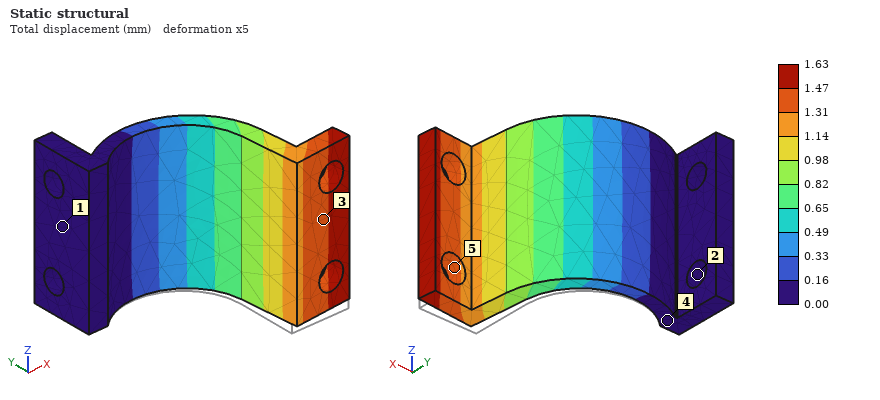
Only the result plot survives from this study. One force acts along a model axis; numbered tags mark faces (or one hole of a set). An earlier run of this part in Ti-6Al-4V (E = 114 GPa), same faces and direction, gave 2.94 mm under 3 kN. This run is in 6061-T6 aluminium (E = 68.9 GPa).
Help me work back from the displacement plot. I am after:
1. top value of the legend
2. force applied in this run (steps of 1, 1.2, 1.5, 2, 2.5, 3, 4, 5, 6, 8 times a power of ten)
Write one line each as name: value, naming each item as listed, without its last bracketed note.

top value of the legend: 1.63 mm
force applied in this run: 1 kN
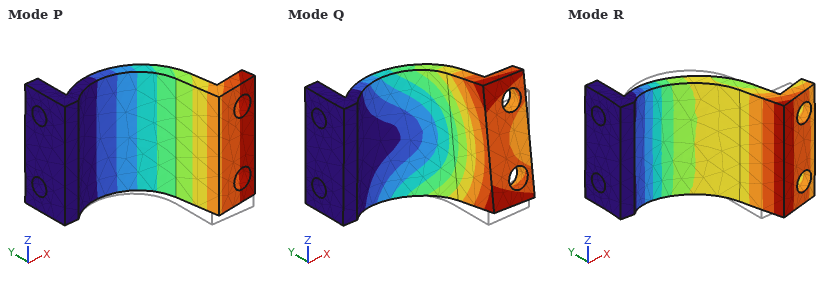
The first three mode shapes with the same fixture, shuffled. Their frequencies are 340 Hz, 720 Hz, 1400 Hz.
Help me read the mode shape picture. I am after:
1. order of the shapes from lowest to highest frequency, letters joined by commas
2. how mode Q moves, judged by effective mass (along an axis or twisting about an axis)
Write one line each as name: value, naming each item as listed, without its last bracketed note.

order of the shapes from lowest to highest frequency, letters joined by commas: P, Q, R
how mode Q moves, judged by effective mass: along Z
